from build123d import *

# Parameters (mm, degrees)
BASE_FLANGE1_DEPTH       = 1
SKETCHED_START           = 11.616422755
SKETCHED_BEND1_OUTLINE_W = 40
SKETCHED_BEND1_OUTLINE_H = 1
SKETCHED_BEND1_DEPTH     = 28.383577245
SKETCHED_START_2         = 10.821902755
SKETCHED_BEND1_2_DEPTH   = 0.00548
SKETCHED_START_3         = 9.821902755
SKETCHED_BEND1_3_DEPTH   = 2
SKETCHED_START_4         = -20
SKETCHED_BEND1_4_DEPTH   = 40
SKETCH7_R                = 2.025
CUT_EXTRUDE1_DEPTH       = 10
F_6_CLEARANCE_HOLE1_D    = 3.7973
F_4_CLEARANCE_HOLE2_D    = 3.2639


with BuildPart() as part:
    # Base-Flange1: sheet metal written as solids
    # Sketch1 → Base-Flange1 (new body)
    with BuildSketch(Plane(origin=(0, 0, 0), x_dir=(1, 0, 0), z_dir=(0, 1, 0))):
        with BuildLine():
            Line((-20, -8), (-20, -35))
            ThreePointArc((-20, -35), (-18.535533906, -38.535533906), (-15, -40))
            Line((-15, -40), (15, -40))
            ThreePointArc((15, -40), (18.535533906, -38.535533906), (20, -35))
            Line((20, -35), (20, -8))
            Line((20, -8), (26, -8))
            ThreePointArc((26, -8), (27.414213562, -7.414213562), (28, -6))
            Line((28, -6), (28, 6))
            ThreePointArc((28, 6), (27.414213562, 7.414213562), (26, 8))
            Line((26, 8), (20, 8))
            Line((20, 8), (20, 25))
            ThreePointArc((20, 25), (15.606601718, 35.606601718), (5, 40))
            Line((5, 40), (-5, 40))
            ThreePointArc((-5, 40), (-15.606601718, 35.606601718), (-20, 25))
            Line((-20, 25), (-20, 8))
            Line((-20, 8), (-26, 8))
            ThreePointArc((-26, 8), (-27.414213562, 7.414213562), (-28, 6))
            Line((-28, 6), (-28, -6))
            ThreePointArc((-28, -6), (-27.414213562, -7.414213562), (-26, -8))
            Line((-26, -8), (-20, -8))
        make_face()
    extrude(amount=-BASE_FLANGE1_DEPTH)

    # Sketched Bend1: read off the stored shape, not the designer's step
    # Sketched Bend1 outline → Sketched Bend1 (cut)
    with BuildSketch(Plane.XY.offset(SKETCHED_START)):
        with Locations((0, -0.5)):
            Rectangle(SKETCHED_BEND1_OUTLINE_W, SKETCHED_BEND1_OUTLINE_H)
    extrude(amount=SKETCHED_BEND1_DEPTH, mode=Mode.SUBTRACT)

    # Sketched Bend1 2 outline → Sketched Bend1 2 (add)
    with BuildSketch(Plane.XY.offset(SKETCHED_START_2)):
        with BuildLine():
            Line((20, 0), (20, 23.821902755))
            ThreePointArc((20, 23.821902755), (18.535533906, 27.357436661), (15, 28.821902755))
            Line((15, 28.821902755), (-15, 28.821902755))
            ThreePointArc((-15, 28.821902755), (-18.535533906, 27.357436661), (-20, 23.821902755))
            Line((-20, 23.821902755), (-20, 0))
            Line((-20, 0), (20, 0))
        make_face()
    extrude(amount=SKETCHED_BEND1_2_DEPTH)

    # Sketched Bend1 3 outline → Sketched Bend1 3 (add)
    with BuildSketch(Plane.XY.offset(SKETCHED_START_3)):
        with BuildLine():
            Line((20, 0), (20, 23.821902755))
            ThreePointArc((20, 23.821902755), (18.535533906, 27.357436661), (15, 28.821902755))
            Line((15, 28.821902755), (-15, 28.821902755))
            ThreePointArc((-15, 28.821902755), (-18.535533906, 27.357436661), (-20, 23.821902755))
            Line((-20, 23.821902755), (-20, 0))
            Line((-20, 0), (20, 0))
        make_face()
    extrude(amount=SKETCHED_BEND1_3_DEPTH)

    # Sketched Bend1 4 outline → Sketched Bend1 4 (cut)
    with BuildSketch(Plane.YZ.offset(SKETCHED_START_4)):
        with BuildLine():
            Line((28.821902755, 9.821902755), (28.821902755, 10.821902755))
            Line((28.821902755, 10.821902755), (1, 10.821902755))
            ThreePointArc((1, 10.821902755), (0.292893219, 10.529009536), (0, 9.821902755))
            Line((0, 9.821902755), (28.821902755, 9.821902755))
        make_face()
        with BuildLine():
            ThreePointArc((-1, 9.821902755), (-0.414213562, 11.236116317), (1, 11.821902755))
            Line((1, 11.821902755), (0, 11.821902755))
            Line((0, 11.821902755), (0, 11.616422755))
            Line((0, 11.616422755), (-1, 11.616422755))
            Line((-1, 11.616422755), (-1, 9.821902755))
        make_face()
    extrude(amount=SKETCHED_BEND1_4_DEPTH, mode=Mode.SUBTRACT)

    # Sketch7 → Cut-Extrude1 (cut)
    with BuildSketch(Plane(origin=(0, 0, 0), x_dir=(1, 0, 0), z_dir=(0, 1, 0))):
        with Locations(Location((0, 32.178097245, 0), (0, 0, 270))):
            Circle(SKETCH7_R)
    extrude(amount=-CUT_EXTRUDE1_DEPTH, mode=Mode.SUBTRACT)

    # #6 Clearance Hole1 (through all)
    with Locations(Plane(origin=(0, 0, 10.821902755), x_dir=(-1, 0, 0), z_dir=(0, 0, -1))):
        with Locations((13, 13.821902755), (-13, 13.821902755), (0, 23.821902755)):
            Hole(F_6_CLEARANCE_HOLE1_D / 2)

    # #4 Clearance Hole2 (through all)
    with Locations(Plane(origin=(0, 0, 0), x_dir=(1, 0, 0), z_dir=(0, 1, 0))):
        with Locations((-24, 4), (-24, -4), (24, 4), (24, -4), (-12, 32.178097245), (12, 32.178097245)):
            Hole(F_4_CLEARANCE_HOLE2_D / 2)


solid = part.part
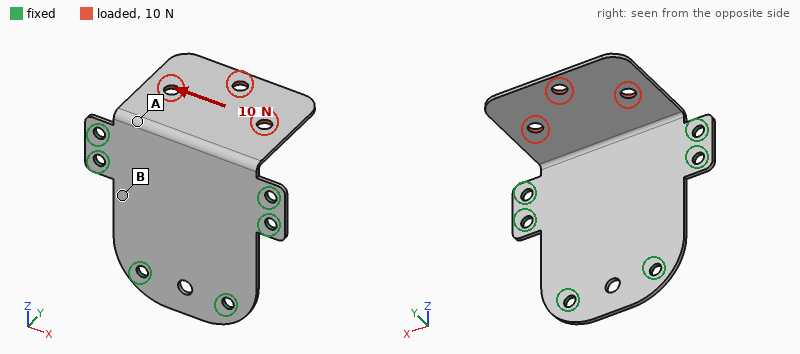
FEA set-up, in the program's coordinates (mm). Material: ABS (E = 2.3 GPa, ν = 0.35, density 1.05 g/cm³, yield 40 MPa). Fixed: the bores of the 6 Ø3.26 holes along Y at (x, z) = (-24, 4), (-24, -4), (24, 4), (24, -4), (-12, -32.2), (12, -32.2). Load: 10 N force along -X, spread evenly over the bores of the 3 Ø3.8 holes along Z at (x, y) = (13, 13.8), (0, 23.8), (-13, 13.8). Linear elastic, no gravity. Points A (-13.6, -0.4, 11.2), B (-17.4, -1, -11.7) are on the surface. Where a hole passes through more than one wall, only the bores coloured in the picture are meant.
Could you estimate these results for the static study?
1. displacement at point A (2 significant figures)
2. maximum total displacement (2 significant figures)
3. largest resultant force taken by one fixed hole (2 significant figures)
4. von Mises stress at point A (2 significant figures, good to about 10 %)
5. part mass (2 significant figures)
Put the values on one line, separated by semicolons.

0.22 mm; 0.71 mm; 6.3 N; 3.8 MPa; 3.4 g
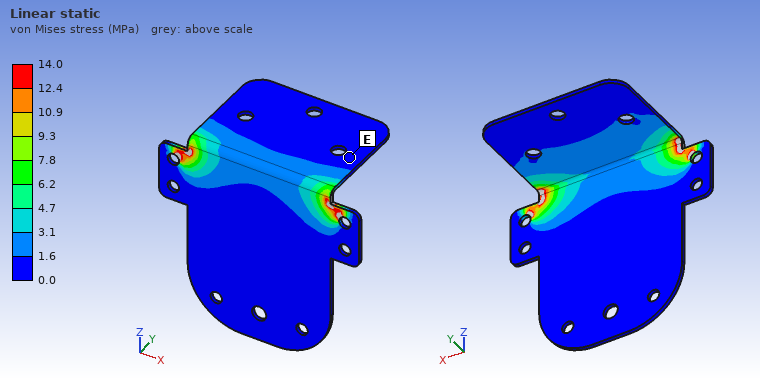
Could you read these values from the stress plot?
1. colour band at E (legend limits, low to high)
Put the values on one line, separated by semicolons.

0.0 to 1.6 MPa
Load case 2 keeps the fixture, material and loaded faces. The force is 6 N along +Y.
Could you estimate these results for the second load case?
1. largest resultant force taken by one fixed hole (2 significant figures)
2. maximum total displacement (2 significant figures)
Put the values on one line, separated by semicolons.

4.1 N; 0.94 mm
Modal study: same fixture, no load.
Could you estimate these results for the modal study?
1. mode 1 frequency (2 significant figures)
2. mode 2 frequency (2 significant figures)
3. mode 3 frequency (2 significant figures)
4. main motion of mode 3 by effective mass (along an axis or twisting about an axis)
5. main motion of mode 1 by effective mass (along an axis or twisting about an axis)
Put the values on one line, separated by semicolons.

200 Hz; 470 Hz; 730 Hz; along Y; along Z
